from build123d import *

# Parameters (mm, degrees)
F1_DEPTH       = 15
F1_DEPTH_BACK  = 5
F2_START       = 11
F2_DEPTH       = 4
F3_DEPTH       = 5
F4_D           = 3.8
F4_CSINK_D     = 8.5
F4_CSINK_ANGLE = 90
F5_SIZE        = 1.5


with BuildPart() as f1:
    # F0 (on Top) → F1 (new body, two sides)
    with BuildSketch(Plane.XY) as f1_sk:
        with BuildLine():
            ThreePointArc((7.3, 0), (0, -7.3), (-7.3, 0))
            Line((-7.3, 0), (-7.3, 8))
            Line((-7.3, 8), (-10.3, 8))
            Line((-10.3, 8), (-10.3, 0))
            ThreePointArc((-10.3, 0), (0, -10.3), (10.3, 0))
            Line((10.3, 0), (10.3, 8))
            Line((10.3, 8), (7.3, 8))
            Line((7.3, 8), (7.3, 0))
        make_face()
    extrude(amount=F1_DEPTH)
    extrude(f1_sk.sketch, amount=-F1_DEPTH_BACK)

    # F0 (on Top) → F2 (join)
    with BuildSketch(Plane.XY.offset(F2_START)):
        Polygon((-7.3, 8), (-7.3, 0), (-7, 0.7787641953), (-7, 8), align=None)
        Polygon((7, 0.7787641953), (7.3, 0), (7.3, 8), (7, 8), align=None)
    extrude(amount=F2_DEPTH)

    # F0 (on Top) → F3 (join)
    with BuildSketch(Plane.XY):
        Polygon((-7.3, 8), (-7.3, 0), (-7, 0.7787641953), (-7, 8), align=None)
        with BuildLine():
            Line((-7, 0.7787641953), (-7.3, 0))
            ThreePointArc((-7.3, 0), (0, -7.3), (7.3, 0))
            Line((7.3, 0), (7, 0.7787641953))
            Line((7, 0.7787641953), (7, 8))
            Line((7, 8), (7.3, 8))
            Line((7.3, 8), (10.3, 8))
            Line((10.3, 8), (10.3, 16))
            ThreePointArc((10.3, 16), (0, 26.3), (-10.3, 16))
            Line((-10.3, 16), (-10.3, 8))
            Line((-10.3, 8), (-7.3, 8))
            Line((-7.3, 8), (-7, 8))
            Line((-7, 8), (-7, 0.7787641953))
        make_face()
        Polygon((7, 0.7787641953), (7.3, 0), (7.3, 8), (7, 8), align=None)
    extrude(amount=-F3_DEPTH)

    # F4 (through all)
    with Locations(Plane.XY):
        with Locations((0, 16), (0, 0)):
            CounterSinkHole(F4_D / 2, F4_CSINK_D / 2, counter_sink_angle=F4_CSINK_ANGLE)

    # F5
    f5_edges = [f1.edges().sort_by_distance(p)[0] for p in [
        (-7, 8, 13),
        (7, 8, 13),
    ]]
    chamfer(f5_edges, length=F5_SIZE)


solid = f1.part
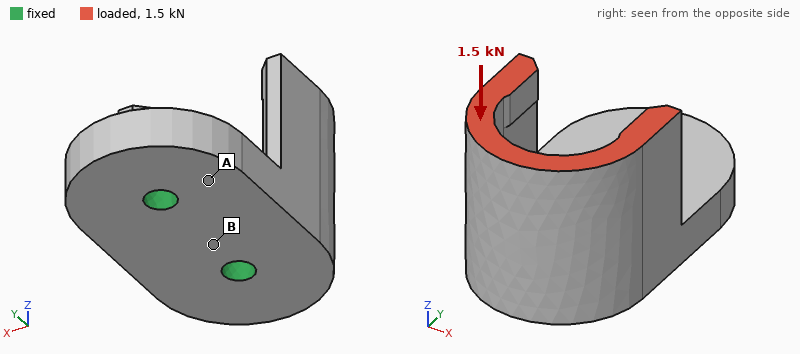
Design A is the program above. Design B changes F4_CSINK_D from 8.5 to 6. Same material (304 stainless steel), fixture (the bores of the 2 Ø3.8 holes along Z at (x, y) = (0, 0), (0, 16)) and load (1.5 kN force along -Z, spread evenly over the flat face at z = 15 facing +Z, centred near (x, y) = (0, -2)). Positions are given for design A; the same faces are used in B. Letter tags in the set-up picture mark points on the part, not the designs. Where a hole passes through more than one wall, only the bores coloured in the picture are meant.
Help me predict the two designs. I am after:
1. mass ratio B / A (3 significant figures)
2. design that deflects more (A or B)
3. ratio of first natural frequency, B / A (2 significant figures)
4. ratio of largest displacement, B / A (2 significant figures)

1.01
A
1.2
0.76
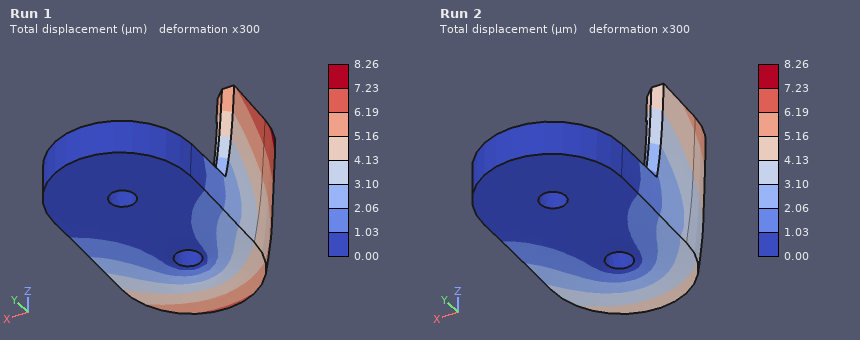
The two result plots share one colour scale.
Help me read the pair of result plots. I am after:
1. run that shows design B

Run 2
